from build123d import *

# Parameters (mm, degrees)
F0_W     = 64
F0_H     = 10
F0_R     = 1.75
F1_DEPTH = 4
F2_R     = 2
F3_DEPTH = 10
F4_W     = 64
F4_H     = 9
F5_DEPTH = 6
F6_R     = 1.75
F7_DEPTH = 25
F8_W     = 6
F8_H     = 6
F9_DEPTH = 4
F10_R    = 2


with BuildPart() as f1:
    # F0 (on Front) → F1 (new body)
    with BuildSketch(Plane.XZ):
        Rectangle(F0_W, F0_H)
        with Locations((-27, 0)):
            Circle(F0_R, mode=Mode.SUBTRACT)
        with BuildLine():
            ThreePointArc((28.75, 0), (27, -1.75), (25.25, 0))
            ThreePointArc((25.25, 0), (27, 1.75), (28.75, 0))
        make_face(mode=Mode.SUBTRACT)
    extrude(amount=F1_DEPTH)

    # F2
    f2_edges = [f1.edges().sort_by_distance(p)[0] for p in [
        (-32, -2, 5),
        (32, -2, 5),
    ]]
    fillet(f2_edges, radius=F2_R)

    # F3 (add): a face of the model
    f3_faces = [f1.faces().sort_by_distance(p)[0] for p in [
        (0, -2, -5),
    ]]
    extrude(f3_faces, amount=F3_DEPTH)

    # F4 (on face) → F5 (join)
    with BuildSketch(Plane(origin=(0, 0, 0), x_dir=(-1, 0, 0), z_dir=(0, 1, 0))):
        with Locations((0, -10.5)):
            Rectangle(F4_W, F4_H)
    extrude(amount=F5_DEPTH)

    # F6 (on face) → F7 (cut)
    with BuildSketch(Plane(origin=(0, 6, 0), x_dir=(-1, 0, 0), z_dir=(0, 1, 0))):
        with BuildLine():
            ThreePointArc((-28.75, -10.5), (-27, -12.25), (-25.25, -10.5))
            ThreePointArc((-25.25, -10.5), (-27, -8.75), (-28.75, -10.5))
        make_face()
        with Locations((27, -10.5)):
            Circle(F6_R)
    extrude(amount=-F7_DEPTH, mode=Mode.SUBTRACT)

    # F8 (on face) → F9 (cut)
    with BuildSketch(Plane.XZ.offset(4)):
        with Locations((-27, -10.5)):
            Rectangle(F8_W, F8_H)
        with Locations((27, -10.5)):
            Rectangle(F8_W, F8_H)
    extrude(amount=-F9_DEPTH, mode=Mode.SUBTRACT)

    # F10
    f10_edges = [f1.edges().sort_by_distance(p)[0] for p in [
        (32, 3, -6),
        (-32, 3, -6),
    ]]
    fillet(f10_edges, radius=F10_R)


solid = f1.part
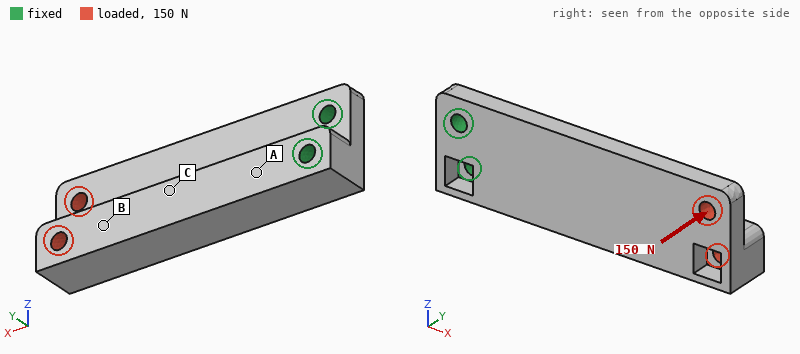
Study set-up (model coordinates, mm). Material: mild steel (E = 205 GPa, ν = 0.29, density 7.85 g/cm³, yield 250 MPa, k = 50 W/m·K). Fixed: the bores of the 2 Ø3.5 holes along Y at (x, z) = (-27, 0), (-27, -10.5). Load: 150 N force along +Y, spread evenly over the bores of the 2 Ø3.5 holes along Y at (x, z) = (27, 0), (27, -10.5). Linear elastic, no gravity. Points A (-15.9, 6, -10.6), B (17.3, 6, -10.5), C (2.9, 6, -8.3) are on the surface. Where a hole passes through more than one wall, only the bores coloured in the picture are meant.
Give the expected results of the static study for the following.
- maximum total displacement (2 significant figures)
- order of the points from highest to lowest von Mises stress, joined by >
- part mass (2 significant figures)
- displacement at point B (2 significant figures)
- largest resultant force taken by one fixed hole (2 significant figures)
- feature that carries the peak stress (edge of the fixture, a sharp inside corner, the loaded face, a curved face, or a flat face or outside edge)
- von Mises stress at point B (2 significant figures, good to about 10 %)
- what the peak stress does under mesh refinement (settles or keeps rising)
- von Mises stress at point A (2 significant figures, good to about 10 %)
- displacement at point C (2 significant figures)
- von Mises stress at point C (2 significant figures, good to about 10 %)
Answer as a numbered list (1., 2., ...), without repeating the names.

1. 70 µm
2. A > C > B
3. 63 g
4. 44 µm
5. 310 N
6. edge of the fixture
7. 9.0 MPa
8. keeps rising
9. 38 MPa
10. 25 µm
11. 24 MPa
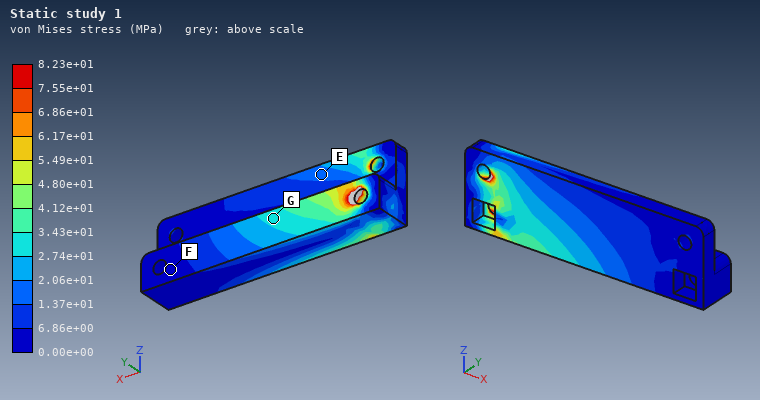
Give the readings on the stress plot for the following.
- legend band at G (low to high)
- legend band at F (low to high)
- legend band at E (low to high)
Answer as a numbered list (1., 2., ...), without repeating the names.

1. 2.74e+01 to 3.43e+01 MPa
2. 0.00e+00 to 6.86e+00 MPa
3. 1.37e+01 to 2.06e+01 MPa
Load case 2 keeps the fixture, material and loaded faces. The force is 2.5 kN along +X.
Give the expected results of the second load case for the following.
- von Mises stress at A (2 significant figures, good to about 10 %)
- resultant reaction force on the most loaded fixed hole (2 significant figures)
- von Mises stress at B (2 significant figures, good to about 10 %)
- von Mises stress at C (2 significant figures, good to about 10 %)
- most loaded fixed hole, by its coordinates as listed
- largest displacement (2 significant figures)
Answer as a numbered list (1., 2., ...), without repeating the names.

1. 34 MPa
2. 1.5 kN
3. 34 MPa
4. 37 MPa
5. (-27, -10.5)
6. 29 µm
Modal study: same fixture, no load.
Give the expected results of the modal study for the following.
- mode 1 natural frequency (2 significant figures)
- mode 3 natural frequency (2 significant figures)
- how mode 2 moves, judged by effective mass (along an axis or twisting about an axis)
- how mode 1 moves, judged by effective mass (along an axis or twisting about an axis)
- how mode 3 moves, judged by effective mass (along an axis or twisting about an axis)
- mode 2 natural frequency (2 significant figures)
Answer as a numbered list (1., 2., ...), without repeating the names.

1. 1800 Hz
2. 7600 Hz
3. along Z
4. along Y
5. twisting about X
6. 4100 Hz
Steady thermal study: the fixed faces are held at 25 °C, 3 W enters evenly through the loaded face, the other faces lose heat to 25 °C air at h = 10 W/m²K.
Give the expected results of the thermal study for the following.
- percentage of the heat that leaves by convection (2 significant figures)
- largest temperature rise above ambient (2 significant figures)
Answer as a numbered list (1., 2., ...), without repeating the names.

1. 15 %
2. 23 K
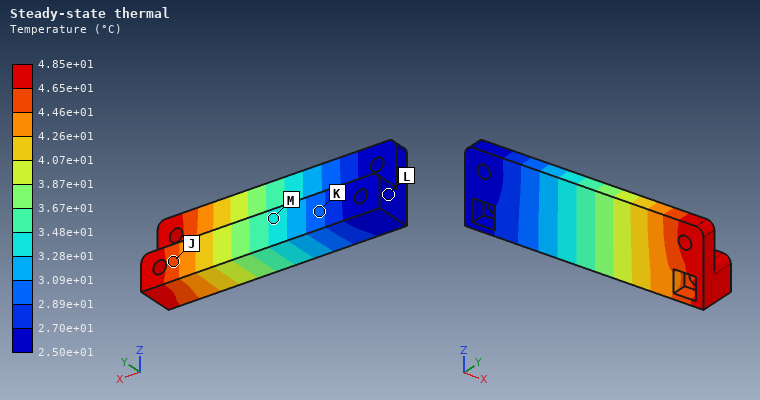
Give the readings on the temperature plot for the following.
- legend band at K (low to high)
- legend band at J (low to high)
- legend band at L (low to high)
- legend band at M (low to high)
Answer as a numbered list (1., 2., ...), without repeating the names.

1. 2.89e+01 to 3.09e+01 °C
2. 4.46e+01 to 4.65e+01 °C
3. 2.50e+01 to 2.70e+01 °C
4. 3.28e+01 to 3.48e+01 °C
